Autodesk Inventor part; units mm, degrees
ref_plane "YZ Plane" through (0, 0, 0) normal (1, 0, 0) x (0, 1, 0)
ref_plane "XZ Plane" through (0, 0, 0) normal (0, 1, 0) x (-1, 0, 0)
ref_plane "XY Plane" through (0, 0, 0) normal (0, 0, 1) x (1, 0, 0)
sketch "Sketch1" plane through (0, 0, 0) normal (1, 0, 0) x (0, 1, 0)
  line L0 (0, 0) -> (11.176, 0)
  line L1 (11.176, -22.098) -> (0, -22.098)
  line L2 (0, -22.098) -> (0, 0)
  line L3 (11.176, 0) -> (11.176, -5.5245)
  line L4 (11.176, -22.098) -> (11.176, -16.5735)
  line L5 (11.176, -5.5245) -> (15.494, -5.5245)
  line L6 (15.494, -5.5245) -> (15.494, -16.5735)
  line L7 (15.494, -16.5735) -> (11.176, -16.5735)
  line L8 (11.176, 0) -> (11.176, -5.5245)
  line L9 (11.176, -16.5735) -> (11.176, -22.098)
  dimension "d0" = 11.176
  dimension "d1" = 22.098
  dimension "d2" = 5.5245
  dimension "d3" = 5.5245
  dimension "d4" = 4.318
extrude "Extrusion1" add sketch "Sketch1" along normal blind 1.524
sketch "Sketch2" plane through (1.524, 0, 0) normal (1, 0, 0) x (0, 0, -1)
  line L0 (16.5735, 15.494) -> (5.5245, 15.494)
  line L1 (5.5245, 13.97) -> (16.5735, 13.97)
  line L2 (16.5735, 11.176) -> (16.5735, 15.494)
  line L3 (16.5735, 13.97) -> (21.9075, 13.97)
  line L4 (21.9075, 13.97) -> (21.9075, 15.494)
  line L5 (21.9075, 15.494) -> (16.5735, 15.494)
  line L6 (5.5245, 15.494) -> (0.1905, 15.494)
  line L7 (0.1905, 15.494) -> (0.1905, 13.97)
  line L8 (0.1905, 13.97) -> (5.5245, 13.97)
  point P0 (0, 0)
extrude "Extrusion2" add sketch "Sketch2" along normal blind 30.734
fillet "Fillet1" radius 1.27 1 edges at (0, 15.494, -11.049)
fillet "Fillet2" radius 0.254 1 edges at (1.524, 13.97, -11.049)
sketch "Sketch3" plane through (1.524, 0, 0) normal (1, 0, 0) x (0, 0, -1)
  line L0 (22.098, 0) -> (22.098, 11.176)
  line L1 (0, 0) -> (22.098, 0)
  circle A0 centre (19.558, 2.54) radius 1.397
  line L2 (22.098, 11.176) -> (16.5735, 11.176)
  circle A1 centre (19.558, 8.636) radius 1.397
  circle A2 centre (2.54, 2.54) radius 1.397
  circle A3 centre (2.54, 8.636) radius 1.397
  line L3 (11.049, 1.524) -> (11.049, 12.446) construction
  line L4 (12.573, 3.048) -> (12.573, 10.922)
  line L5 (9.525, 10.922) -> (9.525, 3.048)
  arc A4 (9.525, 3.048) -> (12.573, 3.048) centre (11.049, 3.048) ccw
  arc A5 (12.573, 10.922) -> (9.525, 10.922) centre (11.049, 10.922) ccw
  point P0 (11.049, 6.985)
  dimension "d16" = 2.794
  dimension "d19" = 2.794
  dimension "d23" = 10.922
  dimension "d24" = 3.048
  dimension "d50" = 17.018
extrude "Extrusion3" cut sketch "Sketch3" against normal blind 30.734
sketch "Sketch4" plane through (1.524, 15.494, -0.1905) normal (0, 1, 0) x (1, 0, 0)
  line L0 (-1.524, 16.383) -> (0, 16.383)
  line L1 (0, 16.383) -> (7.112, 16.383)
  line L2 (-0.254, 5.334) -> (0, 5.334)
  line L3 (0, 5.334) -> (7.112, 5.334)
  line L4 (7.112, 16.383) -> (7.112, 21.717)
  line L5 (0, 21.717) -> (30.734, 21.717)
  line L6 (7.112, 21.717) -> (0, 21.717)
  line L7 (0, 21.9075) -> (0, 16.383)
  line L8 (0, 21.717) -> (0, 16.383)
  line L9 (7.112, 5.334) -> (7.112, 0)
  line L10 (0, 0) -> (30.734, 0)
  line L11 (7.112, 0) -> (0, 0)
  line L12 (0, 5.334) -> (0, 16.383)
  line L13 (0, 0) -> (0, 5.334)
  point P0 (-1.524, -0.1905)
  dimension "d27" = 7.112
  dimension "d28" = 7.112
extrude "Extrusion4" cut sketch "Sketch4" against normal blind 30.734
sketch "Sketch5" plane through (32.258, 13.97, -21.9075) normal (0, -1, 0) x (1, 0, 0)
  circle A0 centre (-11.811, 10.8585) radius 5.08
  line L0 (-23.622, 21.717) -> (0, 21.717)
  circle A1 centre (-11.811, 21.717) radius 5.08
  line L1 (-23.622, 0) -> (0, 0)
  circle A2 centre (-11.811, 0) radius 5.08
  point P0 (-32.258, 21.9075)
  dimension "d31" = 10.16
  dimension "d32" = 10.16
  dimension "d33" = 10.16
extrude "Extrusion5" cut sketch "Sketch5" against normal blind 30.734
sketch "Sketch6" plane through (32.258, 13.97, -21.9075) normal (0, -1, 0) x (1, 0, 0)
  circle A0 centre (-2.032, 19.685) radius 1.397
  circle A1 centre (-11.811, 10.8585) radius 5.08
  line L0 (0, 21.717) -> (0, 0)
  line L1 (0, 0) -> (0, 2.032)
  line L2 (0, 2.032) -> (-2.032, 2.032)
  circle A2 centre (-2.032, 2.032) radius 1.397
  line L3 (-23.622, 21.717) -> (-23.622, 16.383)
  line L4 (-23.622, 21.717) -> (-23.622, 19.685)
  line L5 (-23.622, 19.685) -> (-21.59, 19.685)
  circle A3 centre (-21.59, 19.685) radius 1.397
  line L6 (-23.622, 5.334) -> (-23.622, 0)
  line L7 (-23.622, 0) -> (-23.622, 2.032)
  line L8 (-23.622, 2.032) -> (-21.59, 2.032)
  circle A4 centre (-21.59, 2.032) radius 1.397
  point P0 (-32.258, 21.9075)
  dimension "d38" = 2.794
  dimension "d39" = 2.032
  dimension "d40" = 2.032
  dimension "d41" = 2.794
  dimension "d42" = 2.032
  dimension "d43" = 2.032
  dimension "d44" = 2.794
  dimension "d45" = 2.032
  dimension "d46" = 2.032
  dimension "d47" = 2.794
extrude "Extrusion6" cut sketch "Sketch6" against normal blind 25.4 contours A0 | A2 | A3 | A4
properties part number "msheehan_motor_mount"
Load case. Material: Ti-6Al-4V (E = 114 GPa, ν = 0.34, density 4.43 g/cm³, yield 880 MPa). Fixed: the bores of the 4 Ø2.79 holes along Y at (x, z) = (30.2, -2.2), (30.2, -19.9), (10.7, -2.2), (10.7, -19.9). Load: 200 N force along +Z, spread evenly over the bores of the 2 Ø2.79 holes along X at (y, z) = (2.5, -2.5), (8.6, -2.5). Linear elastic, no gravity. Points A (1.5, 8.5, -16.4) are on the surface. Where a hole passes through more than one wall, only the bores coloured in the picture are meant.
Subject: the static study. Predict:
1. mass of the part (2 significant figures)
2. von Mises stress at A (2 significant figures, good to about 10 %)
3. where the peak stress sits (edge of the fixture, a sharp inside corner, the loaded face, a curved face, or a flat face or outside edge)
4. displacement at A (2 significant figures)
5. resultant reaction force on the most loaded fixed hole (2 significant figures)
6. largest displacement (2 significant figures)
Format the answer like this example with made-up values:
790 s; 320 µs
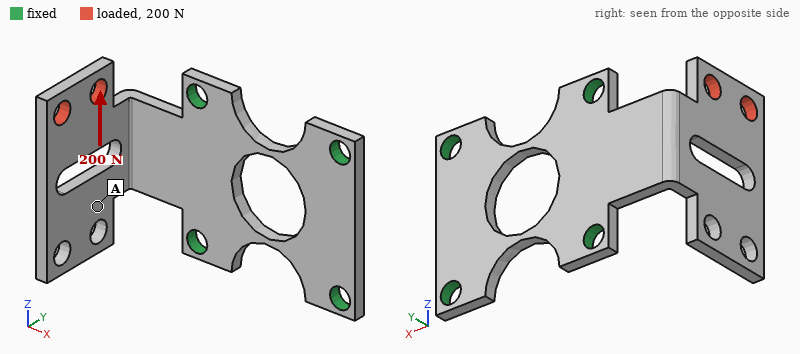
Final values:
4.3 g; 56 MPa; a curved face; 0.20 mm; 230 N; 0.45 mm
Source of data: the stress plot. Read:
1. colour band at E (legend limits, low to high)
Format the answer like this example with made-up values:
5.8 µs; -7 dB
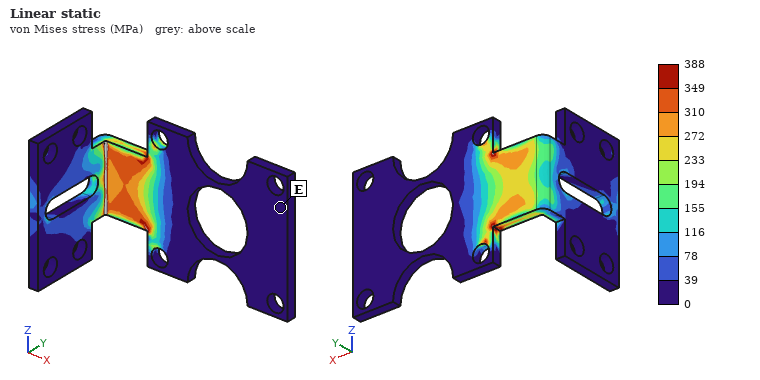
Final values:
0 to 39 MPa
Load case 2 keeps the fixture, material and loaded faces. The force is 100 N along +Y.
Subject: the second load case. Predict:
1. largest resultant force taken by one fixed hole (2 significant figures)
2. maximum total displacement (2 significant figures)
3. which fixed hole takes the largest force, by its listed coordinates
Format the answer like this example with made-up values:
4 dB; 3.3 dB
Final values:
130 N; 0.42 mm; (10.7, -2.2)
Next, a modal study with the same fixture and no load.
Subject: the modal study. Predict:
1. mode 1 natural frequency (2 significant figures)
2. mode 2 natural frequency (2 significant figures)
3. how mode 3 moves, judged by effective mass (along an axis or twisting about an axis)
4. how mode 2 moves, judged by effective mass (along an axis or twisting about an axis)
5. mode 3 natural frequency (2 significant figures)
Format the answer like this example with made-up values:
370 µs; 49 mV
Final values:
2000 Hz; 3200 Hz; along Y; along Z; 5500 Hz
